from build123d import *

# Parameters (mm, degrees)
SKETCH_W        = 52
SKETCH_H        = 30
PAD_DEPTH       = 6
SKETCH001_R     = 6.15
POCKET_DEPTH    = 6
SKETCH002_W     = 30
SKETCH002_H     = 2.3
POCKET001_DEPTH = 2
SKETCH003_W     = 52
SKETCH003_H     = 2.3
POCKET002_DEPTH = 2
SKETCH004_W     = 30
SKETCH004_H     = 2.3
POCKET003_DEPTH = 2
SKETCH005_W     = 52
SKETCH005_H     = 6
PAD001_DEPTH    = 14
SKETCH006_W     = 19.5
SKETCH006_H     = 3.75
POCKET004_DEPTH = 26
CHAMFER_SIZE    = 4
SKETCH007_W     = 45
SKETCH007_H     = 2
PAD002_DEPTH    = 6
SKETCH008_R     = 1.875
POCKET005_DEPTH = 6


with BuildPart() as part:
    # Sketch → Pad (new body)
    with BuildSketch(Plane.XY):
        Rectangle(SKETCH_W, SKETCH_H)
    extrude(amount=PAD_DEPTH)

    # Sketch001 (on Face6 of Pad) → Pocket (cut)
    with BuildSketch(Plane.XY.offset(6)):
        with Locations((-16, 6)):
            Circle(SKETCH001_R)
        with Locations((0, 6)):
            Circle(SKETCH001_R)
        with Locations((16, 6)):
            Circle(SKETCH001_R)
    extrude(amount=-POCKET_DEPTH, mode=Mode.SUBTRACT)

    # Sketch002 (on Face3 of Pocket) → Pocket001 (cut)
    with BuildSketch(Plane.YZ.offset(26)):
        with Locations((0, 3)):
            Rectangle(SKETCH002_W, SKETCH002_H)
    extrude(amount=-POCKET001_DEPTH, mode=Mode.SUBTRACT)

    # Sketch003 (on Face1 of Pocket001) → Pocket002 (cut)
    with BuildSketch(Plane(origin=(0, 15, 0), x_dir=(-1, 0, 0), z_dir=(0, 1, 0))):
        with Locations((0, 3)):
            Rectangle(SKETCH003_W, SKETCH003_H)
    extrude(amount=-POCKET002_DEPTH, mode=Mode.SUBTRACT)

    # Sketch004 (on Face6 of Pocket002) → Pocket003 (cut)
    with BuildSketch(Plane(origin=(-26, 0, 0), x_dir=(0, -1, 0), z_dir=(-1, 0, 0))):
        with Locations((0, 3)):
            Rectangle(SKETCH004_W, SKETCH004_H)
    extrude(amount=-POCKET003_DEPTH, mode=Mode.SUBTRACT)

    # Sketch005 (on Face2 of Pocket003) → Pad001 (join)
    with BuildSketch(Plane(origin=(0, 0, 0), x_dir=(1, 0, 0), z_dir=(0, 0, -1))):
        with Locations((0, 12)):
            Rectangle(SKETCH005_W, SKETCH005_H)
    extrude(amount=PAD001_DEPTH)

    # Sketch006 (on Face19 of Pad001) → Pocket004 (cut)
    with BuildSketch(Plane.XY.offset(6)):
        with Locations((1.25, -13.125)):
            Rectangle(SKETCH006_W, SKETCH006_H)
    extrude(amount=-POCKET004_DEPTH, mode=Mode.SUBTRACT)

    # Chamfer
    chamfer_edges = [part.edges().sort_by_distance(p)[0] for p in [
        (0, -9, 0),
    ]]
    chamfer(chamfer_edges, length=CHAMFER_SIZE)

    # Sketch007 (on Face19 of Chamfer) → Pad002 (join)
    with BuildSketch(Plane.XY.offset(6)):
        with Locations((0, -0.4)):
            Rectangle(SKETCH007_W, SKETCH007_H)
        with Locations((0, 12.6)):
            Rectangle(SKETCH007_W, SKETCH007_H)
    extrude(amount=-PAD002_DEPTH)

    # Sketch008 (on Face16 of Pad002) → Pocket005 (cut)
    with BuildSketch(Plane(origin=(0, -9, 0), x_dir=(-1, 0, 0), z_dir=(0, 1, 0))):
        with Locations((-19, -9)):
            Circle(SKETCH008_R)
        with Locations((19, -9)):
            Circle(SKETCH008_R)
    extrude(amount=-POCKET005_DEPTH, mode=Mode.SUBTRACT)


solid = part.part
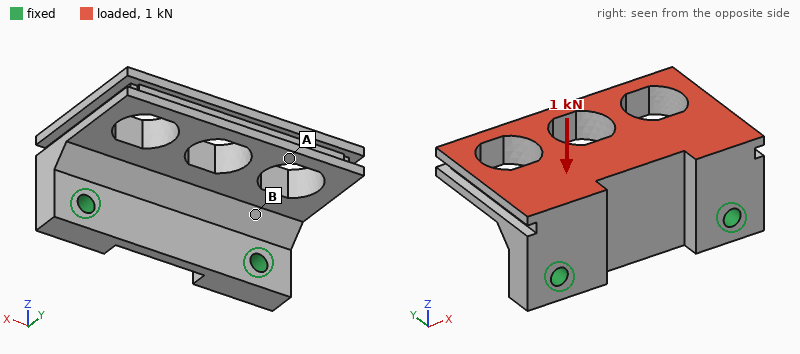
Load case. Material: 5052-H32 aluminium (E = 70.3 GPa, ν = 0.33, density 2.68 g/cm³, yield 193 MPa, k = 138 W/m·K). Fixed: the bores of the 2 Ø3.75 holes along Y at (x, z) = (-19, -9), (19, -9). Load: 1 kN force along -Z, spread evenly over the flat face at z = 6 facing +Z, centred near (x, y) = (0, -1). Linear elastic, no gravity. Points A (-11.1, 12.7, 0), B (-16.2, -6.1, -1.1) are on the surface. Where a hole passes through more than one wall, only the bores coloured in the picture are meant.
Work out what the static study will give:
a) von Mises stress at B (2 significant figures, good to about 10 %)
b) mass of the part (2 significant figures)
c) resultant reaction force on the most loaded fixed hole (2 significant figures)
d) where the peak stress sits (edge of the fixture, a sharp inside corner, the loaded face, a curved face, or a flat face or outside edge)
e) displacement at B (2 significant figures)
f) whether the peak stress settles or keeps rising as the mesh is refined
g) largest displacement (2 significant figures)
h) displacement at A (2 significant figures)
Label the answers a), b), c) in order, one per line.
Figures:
a) 24 MPa
b) 27 g
c) 550 N
d) edge of the fixture
e) 17 µm
f) keeps rising
g) 96 µm
h) 80 µm
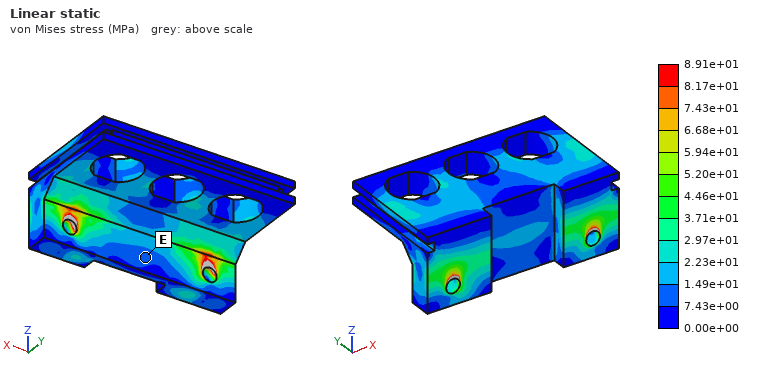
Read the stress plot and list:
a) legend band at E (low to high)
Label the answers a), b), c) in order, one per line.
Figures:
a) 7.43e+00 to 1.49e+01 MPa
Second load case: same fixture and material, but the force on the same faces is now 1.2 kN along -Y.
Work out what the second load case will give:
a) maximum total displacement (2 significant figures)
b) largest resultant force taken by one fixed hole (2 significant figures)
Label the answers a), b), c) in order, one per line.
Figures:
a) 99 µm
b) 600 N
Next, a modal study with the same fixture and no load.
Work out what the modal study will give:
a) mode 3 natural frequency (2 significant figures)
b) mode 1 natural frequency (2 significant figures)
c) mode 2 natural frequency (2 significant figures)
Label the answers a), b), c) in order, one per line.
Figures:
a) 13 kHz
b) 4700 Hz
c) 7700 Hz
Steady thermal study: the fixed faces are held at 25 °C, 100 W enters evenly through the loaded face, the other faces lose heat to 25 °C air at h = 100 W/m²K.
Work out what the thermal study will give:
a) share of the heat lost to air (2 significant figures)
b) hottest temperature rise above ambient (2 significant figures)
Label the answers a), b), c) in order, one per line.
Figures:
a) 16 %
b) 62 K
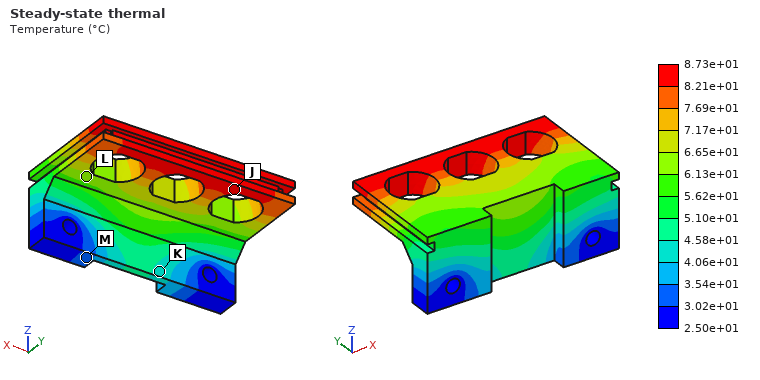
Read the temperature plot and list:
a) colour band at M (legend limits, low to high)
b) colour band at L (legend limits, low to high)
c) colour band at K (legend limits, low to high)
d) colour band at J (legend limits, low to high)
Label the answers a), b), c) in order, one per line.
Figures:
a) 3.02e+01 to 3.54e+01 °C
b) 6.13e+01 to 6.65e+01 °C
c) 4.06e+01 to 4.58e+01 °C
d) 8.21e+01 to 8.73e+01 °C
